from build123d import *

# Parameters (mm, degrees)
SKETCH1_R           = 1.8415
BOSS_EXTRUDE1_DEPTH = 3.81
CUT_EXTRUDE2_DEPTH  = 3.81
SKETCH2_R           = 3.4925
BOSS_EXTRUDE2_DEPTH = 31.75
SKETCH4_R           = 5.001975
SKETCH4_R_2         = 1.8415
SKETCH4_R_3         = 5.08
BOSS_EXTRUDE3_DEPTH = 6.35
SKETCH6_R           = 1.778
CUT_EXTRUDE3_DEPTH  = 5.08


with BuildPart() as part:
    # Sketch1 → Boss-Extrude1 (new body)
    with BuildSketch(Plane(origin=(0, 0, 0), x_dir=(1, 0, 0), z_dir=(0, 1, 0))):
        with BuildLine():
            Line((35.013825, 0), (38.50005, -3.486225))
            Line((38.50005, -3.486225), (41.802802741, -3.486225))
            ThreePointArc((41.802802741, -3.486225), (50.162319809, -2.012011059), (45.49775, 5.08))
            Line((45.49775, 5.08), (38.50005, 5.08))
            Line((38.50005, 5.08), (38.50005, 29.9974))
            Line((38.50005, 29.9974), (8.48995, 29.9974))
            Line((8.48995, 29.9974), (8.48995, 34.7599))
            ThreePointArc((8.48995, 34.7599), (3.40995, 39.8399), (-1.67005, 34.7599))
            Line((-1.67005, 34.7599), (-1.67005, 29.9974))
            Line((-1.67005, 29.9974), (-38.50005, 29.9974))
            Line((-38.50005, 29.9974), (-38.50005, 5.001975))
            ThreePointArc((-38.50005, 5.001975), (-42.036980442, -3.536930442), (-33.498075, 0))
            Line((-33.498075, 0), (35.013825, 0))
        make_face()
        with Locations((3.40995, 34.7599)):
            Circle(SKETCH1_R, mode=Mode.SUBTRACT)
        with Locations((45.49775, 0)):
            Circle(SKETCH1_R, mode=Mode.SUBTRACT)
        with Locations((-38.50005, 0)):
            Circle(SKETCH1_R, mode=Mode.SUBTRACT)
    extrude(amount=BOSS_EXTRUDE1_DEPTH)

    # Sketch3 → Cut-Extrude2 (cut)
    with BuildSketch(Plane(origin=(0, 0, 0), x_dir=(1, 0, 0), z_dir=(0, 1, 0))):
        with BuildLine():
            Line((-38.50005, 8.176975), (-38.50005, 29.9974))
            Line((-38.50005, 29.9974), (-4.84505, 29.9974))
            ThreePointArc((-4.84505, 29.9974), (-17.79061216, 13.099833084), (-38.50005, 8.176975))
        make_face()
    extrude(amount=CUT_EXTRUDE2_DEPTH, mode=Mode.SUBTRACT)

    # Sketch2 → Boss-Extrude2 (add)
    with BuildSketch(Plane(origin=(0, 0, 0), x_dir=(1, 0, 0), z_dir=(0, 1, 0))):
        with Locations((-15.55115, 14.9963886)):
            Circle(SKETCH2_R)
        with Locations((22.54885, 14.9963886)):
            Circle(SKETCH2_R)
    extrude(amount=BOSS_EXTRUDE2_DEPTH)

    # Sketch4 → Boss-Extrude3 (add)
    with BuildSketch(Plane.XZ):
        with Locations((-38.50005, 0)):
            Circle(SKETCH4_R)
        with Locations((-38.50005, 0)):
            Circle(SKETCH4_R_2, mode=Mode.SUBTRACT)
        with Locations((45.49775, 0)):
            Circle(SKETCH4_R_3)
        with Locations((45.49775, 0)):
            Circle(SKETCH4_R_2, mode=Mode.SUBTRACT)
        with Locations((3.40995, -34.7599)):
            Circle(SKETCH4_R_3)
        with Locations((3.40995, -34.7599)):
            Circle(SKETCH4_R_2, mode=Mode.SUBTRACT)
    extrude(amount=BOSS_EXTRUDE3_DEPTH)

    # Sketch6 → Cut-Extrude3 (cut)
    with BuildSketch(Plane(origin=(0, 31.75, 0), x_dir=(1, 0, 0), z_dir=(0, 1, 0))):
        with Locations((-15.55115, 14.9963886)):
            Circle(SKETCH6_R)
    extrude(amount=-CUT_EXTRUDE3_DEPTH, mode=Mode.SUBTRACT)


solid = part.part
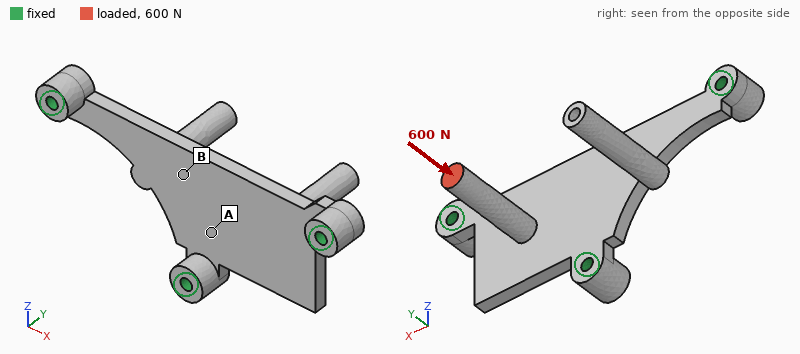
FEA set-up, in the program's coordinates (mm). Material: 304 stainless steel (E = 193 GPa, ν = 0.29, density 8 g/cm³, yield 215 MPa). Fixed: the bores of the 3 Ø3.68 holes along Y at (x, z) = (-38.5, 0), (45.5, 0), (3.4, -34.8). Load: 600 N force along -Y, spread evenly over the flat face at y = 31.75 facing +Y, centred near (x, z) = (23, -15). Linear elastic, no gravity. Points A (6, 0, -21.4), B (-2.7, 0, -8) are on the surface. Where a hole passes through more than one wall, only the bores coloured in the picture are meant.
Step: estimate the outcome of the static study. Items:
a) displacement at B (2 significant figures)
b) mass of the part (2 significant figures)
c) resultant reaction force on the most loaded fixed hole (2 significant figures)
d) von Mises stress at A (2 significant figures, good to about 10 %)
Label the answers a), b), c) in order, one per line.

a) 12 µm
b) 88 g
c) 320 N
d) 19 MPa
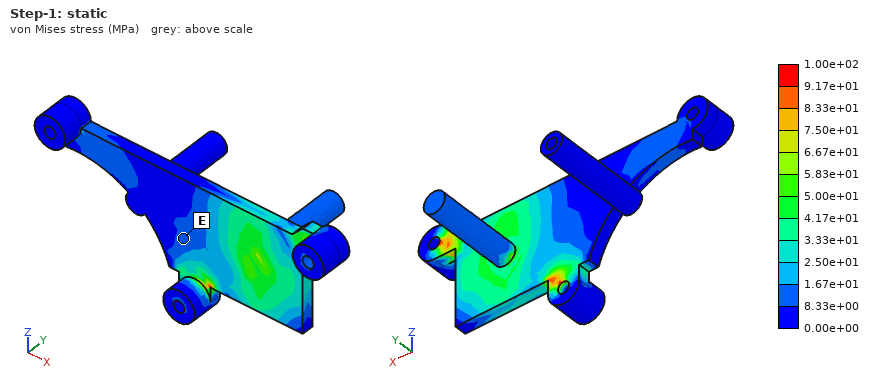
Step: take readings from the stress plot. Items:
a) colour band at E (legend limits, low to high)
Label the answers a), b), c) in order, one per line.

a) 8.33e+00 to 1.67e+01 MPa
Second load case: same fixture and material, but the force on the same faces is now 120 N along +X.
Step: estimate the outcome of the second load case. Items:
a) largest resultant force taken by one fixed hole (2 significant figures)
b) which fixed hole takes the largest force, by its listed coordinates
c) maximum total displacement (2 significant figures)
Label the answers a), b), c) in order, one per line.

a) 89 N
b) (45.5, 0)
c) 78 µm
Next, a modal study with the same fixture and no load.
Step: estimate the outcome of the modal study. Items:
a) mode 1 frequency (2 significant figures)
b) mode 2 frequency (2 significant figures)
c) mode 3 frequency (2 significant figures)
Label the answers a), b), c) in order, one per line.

a) 2500 Hz
b) 3200 Hz
c) 4000 Hz
